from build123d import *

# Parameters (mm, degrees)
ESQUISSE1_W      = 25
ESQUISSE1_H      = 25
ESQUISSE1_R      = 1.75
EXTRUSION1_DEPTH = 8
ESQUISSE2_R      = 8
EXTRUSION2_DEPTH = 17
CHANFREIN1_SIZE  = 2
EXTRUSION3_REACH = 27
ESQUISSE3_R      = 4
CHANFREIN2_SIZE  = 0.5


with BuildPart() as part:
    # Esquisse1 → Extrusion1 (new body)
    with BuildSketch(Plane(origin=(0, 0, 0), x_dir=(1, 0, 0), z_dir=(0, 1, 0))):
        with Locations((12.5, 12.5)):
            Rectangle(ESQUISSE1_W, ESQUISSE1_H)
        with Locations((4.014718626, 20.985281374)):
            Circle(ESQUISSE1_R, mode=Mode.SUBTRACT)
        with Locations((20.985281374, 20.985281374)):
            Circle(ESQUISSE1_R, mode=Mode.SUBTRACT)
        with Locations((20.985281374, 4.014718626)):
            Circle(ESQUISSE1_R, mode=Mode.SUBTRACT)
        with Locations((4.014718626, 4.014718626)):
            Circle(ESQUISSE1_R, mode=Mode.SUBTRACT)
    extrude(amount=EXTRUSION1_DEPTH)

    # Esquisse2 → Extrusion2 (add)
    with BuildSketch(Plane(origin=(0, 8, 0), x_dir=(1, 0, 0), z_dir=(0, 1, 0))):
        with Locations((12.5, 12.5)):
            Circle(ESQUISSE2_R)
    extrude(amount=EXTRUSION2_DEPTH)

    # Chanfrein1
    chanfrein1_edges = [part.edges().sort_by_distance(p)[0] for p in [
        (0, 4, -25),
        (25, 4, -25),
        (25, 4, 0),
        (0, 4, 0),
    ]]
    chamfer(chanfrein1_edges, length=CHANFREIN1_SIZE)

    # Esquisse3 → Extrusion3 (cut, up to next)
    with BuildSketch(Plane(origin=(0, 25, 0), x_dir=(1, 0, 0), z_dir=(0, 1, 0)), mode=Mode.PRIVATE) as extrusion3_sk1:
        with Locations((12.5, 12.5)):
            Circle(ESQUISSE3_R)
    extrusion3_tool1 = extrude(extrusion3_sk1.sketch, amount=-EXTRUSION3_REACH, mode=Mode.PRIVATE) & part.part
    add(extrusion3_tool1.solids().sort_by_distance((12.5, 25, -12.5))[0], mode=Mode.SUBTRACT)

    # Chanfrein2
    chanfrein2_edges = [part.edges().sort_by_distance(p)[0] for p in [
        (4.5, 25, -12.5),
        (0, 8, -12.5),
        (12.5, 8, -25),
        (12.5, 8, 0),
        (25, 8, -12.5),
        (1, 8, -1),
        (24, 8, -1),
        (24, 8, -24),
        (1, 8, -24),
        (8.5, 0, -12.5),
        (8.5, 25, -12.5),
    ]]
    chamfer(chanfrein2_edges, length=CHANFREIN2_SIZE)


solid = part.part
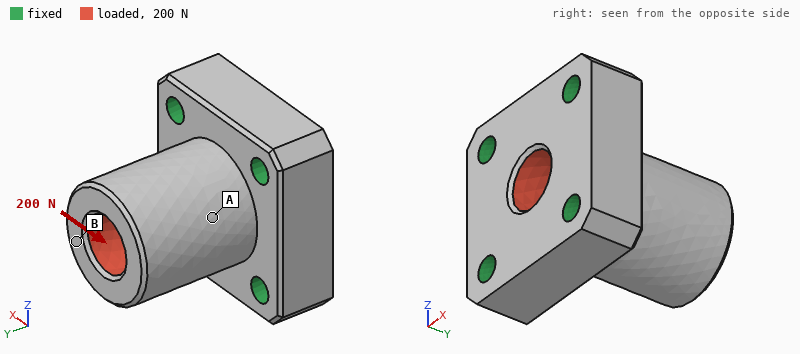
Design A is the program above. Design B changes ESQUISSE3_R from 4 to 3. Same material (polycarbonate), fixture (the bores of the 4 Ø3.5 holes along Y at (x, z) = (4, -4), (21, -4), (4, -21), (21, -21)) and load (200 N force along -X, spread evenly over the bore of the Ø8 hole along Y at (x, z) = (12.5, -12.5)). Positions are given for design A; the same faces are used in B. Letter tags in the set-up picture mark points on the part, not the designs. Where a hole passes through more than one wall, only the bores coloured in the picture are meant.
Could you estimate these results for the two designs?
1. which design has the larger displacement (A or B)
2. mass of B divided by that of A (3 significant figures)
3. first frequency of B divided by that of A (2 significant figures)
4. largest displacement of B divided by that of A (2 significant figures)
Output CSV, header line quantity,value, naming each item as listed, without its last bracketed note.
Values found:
quantity,value
which design has the larger displacement,A
mass of B divided by that of A,1.08
first frequency of B divided by that of A,0.98
largest displacement of B divided by that of A,0.91
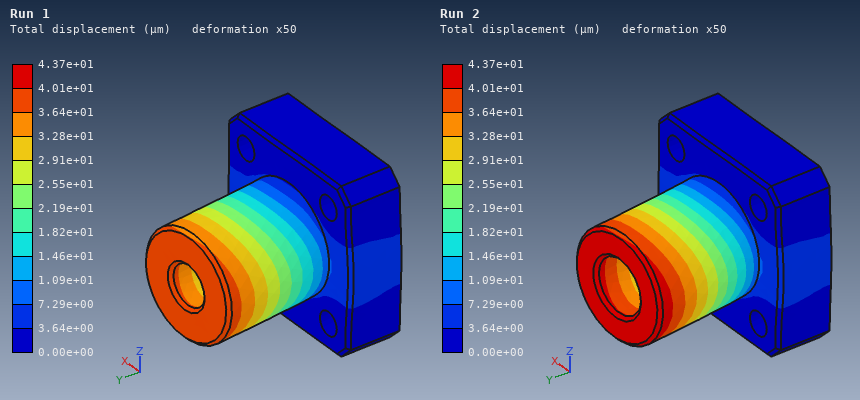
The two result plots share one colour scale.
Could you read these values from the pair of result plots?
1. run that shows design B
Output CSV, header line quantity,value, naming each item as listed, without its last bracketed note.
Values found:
quantity,value
run that shows design B,Run 1
